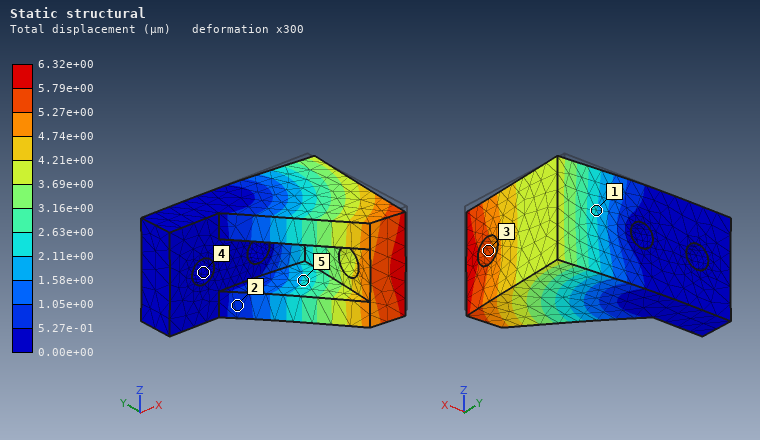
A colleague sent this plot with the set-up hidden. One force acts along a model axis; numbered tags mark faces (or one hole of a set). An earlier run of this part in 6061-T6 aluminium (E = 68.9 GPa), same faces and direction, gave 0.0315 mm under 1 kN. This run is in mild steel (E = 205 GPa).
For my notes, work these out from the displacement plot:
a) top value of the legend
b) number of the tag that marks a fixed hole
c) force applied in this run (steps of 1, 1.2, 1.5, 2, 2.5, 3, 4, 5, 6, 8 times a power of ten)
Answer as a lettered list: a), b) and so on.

a) 6.32e+00 µm
b) 4
c) 600 N
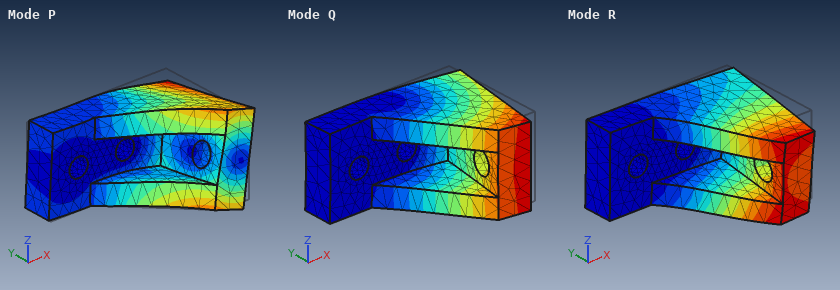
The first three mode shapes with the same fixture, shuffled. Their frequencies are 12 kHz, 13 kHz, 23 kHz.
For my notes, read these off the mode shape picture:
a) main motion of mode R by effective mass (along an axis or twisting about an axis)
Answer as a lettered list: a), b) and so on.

a) along Z
